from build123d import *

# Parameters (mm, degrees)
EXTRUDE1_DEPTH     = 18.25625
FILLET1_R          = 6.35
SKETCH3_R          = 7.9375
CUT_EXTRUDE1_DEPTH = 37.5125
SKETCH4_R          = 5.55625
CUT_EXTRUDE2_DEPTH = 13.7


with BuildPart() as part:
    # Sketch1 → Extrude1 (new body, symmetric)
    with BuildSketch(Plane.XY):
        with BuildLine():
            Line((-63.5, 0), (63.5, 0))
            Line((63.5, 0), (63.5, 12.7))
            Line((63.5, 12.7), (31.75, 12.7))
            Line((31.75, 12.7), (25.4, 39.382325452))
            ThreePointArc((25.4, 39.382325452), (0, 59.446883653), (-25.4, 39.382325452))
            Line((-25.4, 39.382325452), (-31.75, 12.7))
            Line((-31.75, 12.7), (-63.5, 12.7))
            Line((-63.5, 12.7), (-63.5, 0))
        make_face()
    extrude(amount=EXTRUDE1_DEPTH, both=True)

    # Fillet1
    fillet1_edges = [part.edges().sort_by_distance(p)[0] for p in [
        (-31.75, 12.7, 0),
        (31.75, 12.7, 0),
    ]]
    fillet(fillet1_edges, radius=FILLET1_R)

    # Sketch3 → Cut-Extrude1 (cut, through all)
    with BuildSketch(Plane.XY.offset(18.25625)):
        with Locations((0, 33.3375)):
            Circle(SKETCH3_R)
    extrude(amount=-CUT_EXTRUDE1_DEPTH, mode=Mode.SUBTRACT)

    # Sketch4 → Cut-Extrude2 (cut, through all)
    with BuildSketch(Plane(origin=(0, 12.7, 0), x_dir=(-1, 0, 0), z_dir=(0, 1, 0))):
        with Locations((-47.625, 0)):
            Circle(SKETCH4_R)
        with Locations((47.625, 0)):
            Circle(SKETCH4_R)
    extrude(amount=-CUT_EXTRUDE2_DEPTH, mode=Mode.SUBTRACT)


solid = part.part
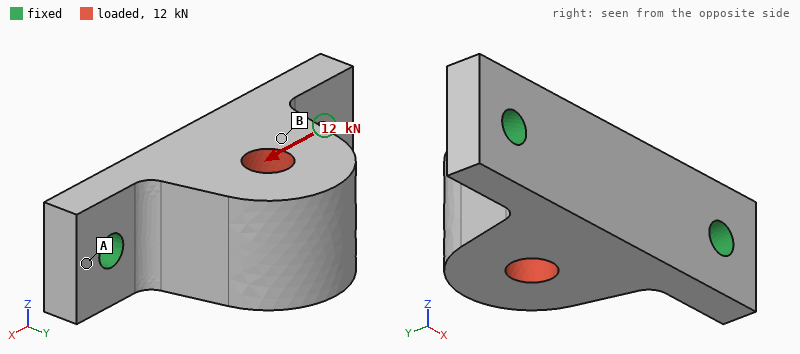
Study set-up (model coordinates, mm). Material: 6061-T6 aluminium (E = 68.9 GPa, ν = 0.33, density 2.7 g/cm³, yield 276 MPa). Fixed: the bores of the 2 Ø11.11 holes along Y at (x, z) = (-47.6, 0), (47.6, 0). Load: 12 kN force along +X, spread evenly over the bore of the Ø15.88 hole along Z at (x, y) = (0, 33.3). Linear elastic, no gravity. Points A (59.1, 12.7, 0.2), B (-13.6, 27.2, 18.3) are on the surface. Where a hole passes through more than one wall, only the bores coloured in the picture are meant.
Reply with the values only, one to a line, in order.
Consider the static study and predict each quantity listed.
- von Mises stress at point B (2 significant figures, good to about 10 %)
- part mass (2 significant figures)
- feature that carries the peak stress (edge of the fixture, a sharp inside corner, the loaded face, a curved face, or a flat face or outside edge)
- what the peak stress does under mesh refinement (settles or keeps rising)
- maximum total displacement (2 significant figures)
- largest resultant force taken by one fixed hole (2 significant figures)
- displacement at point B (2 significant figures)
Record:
12 MPa
360 g
edge of the fixture
keeps rising
27 µm
7.3 kN
14 µm
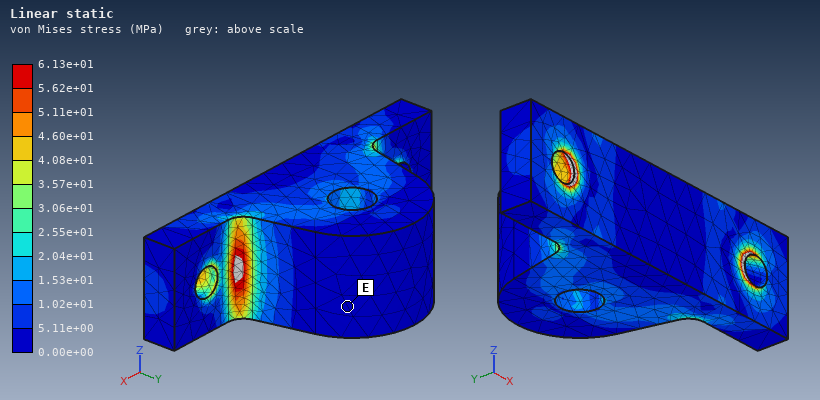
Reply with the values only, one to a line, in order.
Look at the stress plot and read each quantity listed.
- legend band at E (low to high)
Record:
0.00e+00 to 5.11e+00 MPa
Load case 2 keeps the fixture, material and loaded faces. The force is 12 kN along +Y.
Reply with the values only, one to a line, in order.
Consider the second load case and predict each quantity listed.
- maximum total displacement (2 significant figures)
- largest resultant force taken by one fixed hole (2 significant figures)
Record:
28 µm
6.9 kN
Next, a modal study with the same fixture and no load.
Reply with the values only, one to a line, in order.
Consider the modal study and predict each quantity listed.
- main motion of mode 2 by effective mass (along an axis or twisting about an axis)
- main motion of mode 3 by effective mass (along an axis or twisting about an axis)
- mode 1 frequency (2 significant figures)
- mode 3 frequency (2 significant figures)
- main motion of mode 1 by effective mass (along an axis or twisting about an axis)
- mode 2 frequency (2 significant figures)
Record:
along Y
along X
2700 Hz
8000 Hz
along Z
6600 Hz
